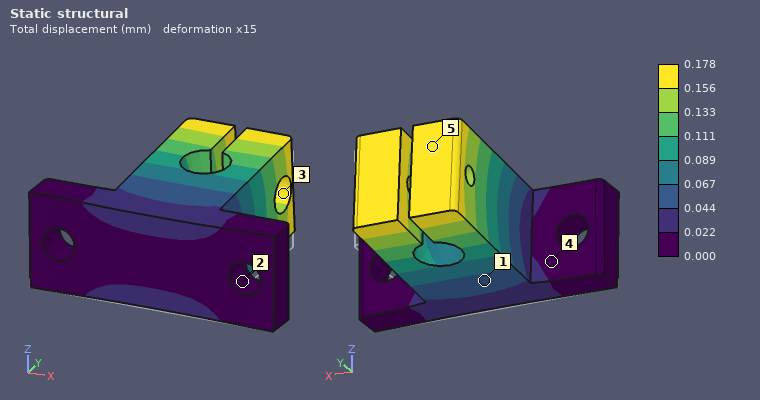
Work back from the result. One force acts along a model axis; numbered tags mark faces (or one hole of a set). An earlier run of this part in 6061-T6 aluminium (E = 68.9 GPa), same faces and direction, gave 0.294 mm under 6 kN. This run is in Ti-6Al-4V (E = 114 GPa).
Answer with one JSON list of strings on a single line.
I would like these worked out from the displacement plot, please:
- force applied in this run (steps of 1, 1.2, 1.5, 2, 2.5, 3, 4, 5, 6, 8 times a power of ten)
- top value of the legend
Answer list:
["6 kN", "0.178 mm"]
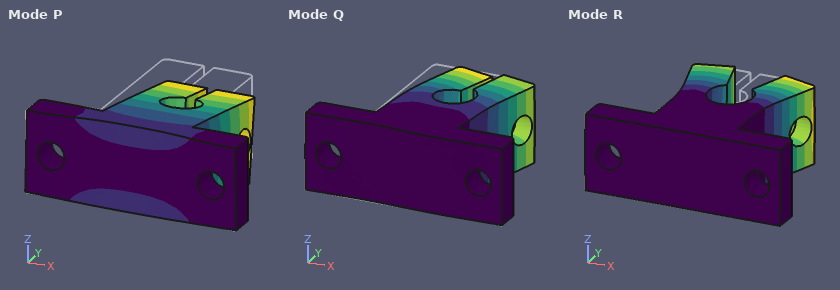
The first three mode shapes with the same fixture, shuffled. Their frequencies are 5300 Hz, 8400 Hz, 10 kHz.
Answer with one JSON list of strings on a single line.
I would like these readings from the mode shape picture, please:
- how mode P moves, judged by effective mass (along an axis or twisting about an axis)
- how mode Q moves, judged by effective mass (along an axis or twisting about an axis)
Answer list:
["along Z", "along X"]
